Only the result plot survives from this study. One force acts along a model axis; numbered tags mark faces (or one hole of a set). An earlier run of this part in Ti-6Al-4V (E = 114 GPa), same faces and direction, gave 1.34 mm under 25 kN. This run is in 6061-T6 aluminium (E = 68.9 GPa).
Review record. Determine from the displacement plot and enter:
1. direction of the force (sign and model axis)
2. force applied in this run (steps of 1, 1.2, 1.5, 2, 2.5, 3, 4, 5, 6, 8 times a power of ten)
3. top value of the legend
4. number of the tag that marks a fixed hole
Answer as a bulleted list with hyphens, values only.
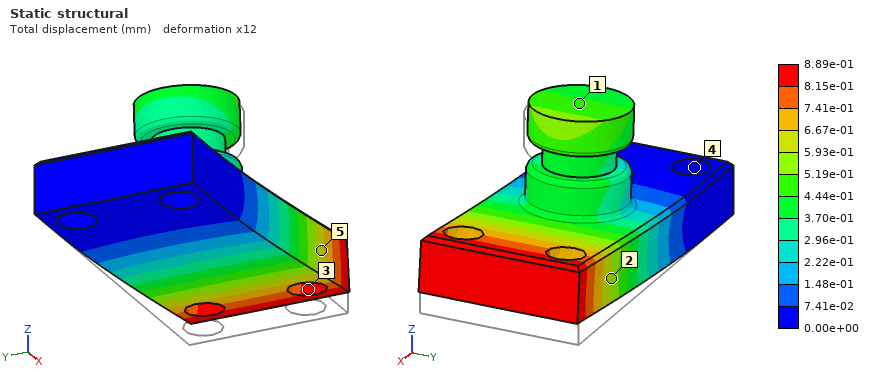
- +Z
- 10 kN
- 8.89e-01 mm
- 4
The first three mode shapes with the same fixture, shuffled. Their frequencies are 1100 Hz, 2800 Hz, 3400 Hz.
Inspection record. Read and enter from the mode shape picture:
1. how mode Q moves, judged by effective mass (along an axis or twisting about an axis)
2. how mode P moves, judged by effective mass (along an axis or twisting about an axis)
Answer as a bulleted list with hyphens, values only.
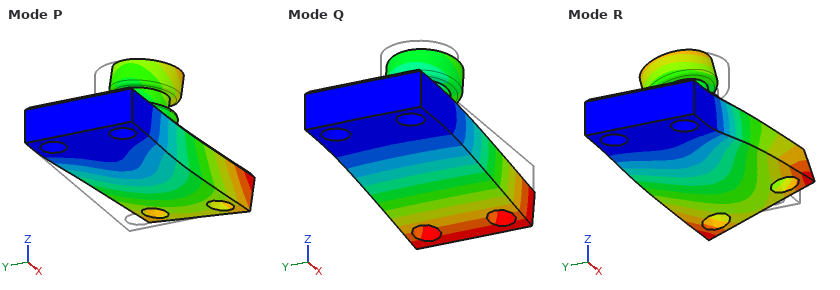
- along Z
- along Y
